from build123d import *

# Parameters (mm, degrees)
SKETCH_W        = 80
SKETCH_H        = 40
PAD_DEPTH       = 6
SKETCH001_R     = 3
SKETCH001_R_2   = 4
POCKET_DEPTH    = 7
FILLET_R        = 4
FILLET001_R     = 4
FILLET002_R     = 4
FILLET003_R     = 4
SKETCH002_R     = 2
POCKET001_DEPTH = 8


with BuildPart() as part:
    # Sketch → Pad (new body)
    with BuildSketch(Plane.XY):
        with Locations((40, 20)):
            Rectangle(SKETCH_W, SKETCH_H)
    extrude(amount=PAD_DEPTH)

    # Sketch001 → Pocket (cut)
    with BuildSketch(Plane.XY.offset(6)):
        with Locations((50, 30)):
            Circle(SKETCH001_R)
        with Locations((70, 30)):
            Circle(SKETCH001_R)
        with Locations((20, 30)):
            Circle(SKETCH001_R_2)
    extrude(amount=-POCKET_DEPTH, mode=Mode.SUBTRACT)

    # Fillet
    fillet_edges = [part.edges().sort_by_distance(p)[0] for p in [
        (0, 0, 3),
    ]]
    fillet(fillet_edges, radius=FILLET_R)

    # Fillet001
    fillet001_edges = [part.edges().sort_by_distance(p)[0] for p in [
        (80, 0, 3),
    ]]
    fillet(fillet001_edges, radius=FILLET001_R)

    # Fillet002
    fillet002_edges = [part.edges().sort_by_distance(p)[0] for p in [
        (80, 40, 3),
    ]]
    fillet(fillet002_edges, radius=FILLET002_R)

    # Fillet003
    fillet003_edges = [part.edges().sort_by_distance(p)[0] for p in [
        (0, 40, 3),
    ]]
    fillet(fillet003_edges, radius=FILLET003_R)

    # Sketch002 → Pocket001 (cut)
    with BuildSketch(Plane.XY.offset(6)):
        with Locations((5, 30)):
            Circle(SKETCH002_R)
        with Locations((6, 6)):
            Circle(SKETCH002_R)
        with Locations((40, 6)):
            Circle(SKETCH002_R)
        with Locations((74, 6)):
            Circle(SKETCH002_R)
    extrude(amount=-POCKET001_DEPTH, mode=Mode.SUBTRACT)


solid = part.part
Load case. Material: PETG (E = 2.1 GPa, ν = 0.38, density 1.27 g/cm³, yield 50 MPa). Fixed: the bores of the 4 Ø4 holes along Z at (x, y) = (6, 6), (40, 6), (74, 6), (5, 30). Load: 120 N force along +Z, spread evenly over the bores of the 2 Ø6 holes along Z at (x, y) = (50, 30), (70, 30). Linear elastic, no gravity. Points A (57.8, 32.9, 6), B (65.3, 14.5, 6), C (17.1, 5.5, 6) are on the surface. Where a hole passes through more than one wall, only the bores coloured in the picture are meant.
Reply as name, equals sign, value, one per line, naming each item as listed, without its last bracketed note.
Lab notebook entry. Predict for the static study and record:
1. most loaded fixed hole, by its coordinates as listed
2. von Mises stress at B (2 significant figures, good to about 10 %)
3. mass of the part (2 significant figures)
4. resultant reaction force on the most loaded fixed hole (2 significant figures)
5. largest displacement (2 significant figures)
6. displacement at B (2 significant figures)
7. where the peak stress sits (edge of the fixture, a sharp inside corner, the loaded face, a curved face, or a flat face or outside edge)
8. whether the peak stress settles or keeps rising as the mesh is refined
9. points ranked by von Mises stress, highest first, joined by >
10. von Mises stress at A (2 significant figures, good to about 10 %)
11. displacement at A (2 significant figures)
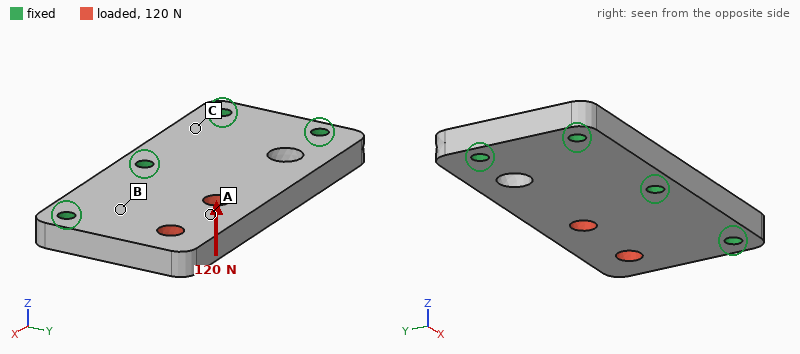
most loaded fixed hole, by its coordinates as listed = (74, 6)
von Mises stress at B = 4.4 MPa
mass of the part = 23 g
resultant reaction force on the most loaded fixed hole = 68 N
largest displacement = 0.57 mm
displacement at B = 0.099 mm
where the peak stress sits = edge of the fixture
whether the peak stress settles or keeps rising as the mesh is refined = keeps rising
points ranked by von Mises stress, highest first, joined by > = B > A > C
von Mises stress at A = 2.7 MPa
displacement at A = 0.38 mm
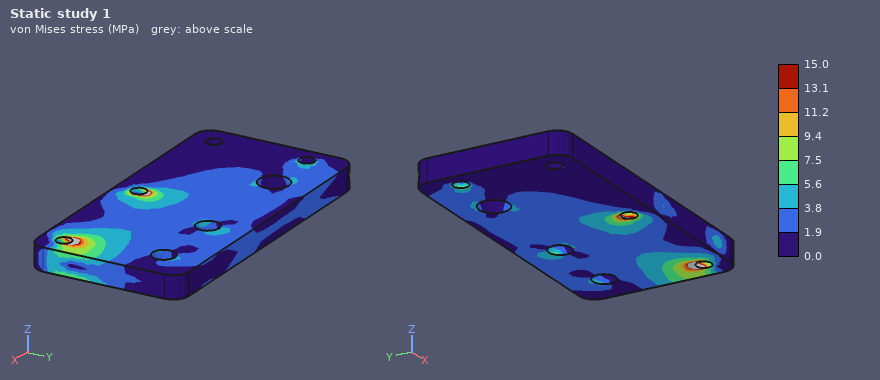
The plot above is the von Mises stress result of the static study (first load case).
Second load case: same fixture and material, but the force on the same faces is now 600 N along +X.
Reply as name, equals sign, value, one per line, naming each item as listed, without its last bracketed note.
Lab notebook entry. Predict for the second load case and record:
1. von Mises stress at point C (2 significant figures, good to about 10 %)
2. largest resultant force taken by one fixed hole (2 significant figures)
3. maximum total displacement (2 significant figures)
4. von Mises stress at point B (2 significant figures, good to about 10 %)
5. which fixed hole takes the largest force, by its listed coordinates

von Mises stress at point C = 0.87 MPa
largest resultant force taken by one fixed hole = 260 N
maximum total displacement = 83 µm
von Mises stress at point B = 2.8 MPa
which fixed hole takes the largest force, by its listed coordinates = (74, 6)
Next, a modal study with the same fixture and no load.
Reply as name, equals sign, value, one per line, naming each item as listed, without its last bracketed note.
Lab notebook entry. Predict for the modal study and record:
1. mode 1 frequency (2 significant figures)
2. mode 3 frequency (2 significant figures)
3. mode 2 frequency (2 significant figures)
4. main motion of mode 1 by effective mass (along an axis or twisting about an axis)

mode 1 frequency = 1100 Hz
mode 3 frequency = 4100 Hz
mode 2 frequency = 2300 Hz
main motion of mode 1 by effective mass = along Z
